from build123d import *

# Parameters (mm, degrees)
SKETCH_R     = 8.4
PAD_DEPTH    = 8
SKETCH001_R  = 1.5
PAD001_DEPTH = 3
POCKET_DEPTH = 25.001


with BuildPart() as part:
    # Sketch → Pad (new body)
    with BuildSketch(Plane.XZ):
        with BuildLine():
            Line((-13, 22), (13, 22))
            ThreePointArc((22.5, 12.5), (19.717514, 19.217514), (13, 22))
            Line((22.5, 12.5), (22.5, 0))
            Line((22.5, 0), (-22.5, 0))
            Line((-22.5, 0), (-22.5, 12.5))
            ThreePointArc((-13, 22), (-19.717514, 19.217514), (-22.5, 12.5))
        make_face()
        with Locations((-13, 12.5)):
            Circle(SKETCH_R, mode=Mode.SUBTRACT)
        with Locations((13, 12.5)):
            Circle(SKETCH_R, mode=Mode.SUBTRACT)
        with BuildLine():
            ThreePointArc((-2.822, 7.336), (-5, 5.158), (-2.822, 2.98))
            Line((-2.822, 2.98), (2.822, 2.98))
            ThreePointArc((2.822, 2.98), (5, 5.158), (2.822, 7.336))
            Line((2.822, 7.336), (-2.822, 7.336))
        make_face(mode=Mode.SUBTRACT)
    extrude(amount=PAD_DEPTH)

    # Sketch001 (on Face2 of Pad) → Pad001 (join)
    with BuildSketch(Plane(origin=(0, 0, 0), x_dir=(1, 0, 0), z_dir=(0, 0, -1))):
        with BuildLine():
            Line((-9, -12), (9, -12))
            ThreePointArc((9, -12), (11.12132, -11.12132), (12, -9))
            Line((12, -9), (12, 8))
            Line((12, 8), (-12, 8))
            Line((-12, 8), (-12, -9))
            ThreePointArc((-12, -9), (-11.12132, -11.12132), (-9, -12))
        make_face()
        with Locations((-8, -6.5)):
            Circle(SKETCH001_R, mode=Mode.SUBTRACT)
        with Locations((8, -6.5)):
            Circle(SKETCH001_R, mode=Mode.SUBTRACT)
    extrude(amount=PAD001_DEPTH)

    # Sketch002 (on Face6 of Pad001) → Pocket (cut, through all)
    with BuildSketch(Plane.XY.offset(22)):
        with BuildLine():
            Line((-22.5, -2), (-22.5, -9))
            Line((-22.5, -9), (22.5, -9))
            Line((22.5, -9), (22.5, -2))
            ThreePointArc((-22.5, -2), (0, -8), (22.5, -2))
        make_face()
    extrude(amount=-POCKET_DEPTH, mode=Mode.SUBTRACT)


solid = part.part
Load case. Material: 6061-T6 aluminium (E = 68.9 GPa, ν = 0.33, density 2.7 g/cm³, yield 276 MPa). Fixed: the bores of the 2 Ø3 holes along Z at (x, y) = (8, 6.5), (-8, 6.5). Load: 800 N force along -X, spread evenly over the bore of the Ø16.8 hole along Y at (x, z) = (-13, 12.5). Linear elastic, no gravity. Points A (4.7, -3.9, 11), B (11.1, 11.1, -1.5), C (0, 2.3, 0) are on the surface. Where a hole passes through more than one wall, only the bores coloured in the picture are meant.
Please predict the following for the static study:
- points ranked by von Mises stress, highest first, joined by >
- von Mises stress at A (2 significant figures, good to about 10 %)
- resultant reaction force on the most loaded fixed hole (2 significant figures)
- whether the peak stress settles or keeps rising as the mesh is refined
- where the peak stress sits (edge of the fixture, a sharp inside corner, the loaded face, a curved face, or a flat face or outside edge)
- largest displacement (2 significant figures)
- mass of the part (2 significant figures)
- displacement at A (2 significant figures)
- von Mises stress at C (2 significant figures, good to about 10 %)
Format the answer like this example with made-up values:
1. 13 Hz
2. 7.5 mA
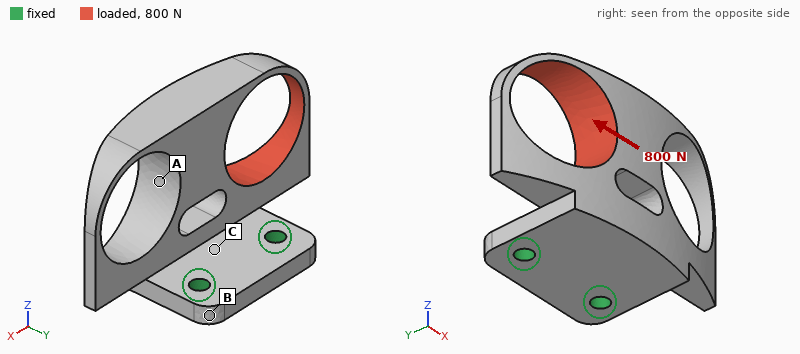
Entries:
1. C > A > B
2. 36 MPa
3. 860 N
4. keeps rising
5. edge of the fixture
6. 0.14 mm
7. 12 g
8. 0.054 mm
9. 71 MPa
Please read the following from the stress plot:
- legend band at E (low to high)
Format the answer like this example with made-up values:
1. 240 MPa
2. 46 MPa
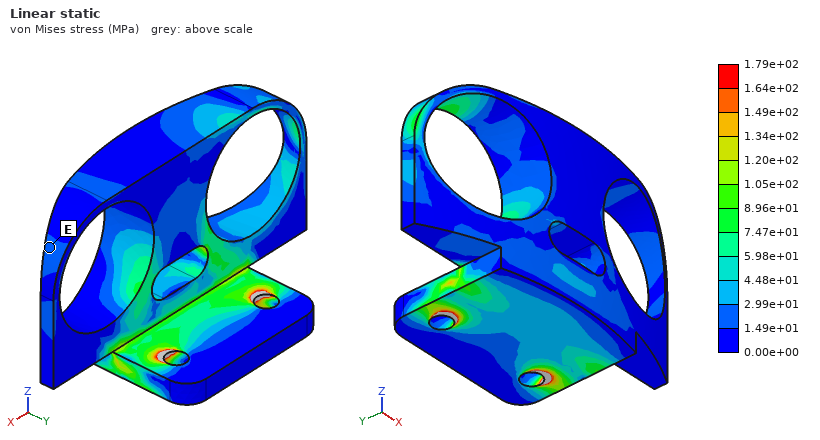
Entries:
1. 1.49e+01 to 2.99e+01 MPa
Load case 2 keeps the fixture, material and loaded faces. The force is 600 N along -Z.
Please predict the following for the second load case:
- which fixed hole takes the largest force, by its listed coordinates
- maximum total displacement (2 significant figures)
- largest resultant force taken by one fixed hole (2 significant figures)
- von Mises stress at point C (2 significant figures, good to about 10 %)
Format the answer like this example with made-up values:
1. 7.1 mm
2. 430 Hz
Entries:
1. (-8, 6.5)
2. 0.23 mm
3. 680 N
4. 69 MPa
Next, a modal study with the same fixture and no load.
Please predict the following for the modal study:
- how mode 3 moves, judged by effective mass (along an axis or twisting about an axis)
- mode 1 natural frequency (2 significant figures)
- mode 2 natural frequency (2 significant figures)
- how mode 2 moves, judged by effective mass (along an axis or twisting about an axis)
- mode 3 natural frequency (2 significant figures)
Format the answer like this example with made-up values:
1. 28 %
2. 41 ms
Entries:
1. along Z
2. 2400 Hz
3. 5600 Hz
4. along X
5. 10000 Hz
